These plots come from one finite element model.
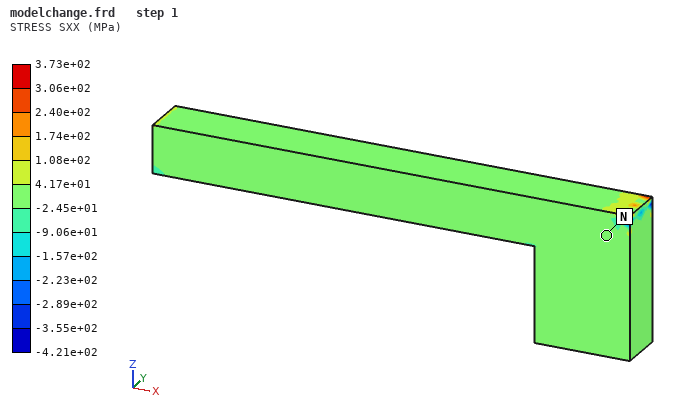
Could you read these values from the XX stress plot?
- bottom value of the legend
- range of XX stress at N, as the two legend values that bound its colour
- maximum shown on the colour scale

-4.21e+02 MPa
-2.45e+01 to 4.17e+01 MPa
3.73e+02 MPa
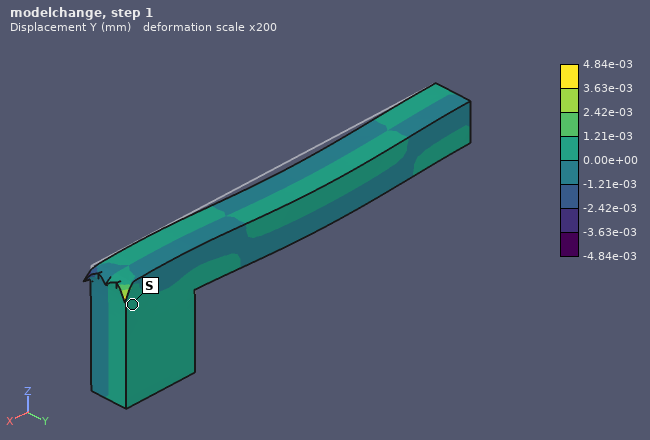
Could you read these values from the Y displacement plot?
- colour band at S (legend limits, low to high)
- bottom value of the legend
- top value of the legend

0.00e+00 to 1.21e-03 mm
-4.84e-03 mm
4.84e-03 mm
